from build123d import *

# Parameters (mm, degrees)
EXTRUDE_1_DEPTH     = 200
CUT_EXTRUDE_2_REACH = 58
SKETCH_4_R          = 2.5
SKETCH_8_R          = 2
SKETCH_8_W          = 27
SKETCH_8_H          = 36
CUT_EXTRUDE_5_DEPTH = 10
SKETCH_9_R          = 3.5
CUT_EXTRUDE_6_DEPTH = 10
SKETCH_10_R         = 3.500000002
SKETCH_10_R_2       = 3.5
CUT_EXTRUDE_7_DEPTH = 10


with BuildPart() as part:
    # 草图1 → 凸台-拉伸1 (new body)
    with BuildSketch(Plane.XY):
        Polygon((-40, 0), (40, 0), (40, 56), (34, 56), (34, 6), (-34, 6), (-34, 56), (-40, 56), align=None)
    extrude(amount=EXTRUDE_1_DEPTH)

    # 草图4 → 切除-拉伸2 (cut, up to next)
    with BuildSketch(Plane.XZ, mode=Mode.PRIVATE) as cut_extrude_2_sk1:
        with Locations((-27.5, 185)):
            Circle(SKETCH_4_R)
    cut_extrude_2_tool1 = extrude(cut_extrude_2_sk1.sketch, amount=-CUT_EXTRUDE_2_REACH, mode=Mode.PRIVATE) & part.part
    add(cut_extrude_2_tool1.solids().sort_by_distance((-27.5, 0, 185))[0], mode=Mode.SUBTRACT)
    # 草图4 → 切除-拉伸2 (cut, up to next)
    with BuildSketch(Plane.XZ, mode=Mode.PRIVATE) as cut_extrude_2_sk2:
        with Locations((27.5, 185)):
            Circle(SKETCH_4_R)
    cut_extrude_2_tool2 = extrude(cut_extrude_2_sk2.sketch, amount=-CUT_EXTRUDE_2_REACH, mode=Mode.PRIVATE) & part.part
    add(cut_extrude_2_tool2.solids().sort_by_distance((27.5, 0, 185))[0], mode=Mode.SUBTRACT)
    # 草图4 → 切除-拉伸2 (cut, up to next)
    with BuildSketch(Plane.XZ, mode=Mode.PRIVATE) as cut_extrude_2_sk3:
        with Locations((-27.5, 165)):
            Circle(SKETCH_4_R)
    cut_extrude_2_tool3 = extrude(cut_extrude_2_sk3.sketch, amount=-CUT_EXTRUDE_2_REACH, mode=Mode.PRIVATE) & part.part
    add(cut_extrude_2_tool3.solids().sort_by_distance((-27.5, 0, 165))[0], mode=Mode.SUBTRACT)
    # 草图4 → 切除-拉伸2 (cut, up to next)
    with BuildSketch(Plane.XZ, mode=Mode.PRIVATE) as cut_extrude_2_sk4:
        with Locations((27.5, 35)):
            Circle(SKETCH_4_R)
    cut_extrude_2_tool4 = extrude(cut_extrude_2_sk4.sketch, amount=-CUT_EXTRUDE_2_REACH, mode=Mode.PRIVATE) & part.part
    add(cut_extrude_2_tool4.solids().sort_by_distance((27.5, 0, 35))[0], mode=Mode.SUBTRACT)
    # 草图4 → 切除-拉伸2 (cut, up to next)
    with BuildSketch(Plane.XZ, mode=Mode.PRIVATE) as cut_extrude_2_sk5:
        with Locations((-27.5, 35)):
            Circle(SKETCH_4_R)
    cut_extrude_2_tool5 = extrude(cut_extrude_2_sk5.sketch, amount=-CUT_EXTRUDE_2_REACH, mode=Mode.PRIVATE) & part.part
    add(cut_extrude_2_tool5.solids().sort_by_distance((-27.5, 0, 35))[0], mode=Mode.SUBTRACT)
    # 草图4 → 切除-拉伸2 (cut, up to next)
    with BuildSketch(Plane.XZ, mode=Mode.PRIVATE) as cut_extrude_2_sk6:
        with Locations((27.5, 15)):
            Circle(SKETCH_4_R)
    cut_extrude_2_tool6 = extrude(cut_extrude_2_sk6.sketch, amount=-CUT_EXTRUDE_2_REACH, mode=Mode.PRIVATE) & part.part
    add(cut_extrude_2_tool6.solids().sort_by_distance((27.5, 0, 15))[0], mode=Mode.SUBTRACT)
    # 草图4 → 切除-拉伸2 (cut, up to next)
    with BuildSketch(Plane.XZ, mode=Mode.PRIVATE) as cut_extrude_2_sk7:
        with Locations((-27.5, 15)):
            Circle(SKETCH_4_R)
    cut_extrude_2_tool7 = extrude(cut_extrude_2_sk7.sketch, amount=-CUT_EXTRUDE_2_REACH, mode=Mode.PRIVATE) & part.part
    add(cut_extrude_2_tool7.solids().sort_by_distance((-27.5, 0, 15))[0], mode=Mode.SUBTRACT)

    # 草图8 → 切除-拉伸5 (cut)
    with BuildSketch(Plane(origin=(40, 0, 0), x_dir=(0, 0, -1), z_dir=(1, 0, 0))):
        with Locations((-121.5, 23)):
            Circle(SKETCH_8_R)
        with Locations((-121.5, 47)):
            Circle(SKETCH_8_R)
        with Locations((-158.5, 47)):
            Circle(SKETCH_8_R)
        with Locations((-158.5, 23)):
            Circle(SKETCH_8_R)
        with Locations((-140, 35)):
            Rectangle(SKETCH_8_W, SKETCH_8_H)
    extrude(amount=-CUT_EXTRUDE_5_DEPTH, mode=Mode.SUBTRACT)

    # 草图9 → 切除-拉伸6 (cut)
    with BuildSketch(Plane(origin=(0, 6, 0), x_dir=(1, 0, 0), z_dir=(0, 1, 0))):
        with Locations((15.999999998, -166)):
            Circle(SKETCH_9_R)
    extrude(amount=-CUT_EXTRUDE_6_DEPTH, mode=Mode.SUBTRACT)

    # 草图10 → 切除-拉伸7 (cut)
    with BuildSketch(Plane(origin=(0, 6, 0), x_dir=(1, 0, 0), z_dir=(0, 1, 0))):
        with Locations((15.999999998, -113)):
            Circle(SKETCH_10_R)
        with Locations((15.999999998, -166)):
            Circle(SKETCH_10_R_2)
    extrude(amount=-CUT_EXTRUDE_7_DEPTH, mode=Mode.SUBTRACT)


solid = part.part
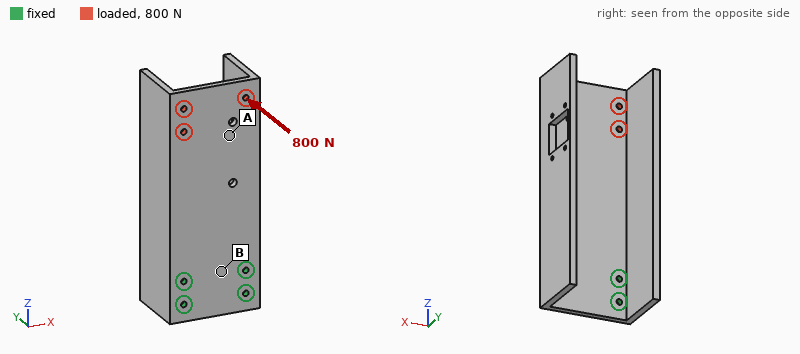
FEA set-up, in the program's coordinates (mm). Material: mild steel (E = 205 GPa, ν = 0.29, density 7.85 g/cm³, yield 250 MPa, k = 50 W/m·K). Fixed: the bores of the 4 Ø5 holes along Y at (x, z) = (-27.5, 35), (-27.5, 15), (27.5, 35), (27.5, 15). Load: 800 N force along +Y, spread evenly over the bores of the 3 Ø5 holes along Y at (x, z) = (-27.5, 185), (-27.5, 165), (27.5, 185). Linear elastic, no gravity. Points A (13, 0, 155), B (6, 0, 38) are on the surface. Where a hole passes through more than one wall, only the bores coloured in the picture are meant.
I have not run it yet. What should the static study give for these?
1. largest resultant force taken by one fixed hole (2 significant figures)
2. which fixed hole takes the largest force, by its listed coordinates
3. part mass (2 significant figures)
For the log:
3.0 kN
(-27.5, 35)
1.6 kg
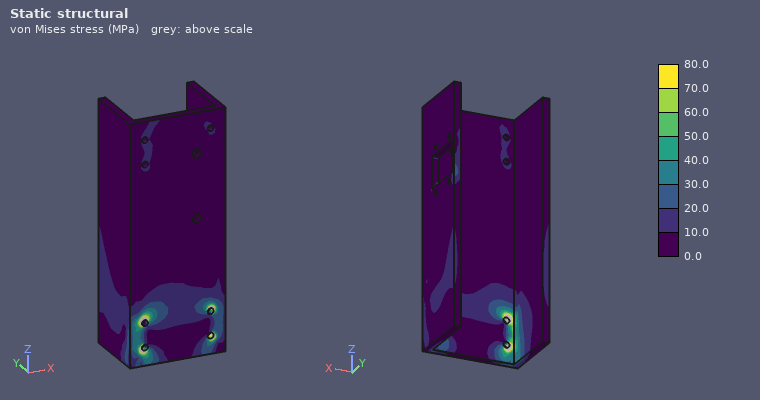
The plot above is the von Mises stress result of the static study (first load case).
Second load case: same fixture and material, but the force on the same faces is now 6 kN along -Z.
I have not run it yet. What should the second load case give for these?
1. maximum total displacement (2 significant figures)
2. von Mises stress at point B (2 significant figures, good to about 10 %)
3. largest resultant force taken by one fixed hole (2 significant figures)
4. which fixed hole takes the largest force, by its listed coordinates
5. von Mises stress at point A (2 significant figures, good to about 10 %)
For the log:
28 µm
5.6 MPa
2.7 kN
(-27.5, 35)
6.3 MPa
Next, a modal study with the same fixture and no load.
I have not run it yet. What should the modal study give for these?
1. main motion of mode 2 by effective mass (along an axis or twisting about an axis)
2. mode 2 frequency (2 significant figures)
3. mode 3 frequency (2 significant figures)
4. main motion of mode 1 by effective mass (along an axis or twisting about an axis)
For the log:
along X
600 Hz
1100 Hz
along Y
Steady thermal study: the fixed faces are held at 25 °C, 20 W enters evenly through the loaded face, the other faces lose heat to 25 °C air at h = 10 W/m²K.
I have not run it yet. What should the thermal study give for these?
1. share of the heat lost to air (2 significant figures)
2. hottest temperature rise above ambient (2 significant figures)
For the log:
61 %
46 K
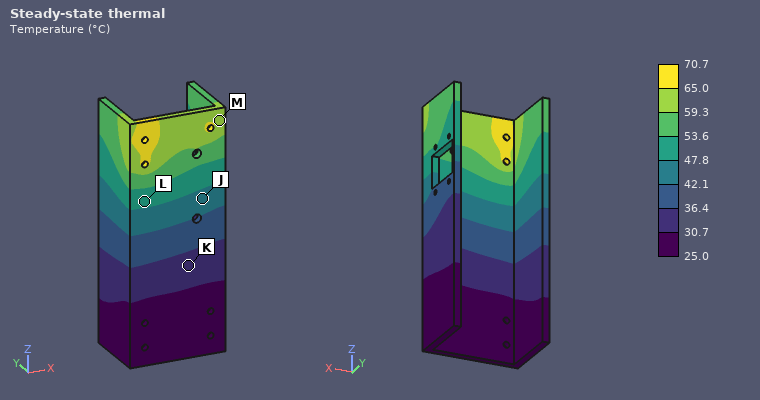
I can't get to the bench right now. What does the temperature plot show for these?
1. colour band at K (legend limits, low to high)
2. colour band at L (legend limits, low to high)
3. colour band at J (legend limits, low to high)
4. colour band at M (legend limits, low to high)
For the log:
30.7 to 36.4 °C
47.8 to 53.6 °C
42.1 to 47.8 °C
59.3 to 65.0 °C
